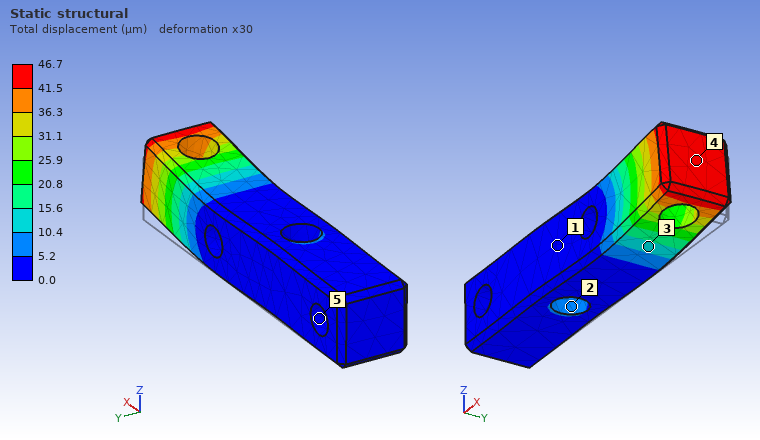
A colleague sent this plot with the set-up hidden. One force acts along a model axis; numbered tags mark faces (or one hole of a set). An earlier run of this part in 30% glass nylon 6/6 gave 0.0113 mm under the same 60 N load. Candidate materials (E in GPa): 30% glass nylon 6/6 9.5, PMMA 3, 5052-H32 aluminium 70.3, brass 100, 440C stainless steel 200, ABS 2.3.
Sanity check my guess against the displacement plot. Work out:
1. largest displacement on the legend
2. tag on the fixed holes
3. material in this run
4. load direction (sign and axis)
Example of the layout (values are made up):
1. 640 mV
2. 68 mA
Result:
1. 46.7 µm
2. 5
3. ABS
4. +Z
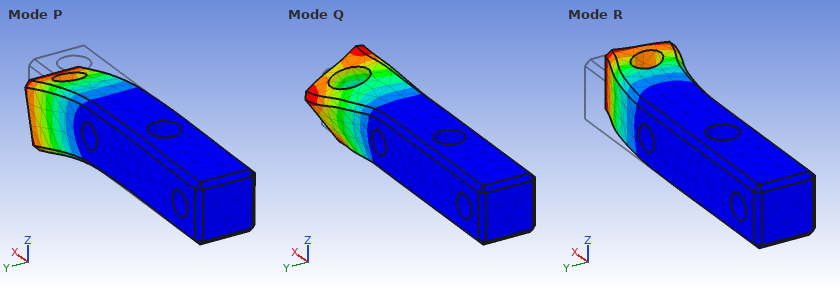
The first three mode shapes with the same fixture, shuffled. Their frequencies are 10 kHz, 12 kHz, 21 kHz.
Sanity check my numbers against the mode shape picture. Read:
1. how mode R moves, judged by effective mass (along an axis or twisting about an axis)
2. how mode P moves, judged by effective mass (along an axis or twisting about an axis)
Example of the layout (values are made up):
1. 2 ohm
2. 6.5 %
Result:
1. along Y
2. along Z
